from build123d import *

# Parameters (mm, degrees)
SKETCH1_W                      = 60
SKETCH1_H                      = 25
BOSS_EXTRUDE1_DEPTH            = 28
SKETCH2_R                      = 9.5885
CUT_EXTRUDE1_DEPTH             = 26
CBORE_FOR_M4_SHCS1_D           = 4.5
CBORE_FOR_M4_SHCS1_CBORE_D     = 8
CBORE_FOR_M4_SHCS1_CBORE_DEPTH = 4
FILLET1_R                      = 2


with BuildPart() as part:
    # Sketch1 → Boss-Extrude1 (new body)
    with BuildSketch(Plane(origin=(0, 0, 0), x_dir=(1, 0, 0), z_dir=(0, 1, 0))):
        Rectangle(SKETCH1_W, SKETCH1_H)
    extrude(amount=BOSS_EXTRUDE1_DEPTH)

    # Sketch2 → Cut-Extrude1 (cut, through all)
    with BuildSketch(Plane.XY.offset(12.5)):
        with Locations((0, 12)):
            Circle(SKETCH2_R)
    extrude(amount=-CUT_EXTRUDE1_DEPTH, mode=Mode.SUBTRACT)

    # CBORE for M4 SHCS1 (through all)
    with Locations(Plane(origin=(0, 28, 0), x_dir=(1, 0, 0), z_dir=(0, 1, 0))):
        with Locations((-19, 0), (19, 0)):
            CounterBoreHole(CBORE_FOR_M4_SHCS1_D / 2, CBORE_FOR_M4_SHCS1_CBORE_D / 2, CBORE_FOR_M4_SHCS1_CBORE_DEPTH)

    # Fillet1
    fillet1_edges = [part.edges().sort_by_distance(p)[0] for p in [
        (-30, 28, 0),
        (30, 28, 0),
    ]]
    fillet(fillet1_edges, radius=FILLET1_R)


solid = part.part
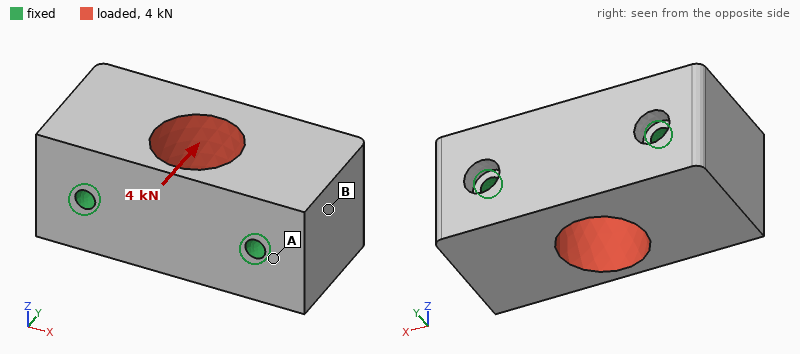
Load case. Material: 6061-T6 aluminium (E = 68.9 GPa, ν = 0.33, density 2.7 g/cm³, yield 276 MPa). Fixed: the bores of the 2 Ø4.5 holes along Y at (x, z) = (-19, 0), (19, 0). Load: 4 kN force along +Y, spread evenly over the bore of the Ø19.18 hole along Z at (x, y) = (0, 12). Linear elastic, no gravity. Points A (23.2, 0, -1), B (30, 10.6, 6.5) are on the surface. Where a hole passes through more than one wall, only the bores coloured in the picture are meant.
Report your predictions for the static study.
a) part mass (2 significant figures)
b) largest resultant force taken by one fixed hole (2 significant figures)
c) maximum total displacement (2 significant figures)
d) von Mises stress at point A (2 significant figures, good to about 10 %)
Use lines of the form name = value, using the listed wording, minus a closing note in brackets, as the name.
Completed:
part mass = 91 g
largest resultant force taken by one fixed hole = 2.0 kN
maximum total displacement = 5.7 µm
von Mises stress at point A = 4.7 MPa
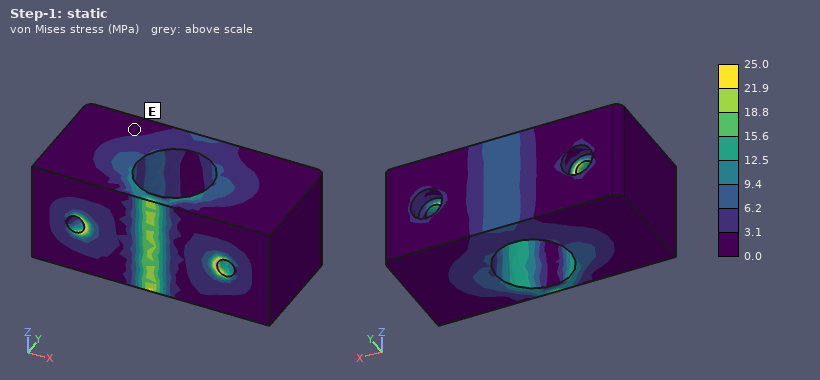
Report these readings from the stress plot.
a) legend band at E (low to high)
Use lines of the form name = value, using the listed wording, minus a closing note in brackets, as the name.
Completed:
legend band at E = 0.0 to 3.1 MPa
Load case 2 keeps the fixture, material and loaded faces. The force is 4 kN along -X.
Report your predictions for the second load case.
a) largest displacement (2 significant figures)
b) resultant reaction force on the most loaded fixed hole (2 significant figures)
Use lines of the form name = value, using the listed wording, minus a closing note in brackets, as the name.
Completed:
largest displacement = 1.4 µm
resultant reaction force on the most loaded fixed hole = 2.0 kN
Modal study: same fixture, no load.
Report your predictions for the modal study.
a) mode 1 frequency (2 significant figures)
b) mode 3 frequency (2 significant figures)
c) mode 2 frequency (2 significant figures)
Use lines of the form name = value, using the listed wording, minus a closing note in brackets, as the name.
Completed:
mode 1 frequency = 23 kHz
mode 3 frequency = 31 kHz
mode 2 frequency = 30 kHz
